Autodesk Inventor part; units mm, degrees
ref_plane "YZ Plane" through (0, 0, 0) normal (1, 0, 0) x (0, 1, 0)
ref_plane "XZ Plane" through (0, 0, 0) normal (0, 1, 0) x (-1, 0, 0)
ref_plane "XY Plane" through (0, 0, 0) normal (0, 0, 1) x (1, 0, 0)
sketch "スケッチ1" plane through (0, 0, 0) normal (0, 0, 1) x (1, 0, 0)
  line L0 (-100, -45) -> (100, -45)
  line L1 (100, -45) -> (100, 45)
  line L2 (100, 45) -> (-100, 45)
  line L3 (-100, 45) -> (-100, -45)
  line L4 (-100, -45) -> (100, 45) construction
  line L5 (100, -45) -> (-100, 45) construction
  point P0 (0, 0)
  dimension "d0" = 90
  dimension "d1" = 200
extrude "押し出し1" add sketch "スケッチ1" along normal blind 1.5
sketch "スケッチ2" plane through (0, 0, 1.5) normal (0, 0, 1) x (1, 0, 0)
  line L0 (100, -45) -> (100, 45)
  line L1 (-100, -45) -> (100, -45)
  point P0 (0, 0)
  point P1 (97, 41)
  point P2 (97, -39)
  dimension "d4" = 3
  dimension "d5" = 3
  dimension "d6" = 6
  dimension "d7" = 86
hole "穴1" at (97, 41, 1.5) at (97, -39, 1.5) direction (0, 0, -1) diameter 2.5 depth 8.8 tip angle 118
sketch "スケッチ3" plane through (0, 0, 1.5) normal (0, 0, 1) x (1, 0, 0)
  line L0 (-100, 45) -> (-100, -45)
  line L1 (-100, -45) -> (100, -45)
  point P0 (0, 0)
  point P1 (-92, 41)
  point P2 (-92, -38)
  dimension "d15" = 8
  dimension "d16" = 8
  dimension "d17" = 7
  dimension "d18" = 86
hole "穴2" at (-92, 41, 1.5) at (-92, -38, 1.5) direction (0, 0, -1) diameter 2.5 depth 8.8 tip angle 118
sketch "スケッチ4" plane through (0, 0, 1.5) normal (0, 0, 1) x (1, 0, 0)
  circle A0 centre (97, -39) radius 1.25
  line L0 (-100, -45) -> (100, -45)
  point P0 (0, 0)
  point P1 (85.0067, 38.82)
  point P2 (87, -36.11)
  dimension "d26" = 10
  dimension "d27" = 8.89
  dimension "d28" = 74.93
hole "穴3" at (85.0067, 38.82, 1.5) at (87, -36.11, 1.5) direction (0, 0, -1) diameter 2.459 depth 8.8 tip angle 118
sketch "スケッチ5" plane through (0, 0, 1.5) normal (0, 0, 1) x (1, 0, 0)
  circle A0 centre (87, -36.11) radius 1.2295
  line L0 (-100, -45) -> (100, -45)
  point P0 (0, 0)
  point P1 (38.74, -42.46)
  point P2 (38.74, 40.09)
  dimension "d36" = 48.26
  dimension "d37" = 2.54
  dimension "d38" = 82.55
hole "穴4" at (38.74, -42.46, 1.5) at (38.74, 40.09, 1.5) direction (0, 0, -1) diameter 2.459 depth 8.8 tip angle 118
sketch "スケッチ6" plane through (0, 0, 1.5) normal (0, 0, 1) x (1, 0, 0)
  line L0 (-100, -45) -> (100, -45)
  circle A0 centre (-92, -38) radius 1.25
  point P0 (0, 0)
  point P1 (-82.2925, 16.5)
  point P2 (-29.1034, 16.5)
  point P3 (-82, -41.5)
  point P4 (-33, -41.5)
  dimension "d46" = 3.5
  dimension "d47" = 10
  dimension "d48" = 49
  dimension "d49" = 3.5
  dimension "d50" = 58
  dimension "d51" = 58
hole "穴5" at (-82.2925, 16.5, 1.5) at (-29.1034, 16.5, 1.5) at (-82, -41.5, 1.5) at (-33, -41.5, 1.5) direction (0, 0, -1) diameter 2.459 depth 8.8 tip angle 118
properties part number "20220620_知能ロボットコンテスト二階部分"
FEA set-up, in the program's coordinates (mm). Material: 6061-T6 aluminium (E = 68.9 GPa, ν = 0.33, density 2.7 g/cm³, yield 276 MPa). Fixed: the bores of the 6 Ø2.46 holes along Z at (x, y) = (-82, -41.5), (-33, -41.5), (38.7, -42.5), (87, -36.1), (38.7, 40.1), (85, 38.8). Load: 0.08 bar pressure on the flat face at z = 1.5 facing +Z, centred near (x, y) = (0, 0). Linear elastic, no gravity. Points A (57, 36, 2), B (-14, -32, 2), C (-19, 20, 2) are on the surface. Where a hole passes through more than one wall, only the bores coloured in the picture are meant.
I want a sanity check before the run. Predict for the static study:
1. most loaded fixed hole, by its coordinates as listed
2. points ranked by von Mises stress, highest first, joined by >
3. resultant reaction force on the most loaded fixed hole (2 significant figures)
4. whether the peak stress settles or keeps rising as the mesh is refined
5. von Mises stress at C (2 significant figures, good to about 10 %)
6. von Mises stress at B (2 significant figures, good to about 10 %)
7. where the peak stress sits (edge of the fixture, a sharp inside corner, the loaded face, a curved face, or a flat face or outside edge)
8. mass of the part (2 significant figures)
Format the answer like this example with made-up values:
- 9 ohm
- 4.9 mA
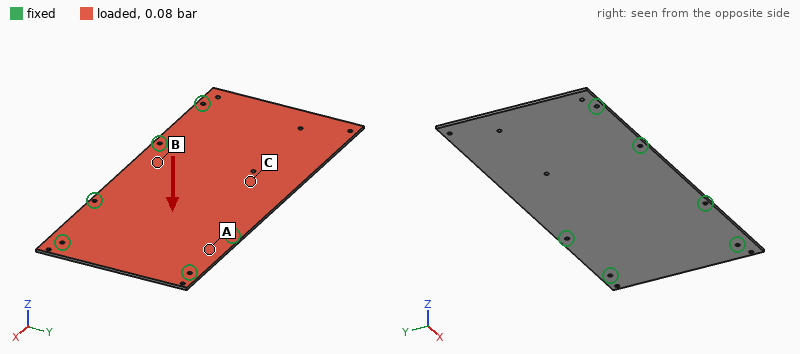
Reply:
- (38.7, 40.1)
- C > B > A
- 45 N
- keeps rising
- 24 MPa
- 14 MPa
- edge of the fixture
- 73 g
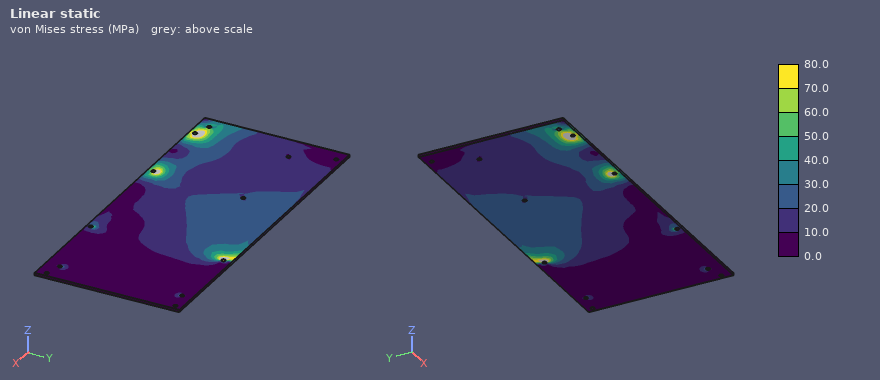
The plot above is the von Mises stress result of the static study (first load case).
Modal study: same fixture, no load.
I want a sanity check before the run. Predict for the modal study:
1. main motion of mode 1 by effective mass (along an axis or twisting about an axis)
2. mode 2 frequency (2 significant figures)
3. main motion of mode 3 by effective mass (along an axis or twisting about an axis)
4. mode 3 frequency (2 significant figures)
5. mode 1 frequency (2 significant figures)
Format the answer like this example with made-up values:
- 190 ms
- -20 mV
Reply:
- along Z
- 530 Hz
- along Z
- 900 Hz
- 210 Hz
